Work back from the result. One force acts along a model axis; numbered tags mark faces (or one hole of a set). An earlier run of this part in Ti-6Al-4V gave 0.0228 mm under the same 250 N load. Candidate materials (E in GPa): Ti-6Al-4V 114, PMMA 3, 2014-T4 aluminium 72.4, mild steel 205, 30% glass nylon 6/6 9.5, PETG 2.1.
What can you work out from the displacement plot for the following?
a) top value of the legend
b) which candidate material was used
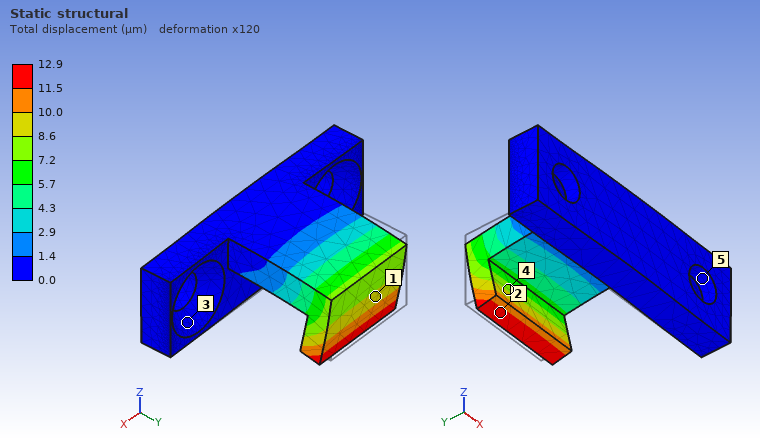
12.9 µm
mild steel
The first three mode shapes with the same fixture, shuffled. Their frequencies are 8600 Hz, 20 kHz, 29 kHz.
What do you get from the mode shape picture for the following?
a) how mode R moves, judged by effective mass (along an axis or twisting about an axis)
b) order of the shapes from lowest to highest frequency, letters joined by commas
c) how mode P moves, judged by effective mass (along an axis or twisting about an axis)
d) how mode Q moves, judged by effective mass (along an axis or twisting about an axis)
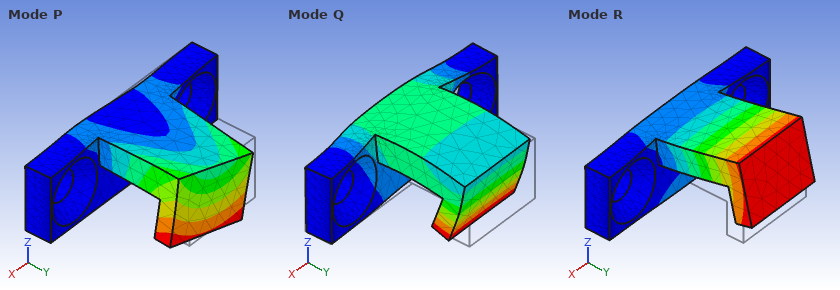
along Z
R, P, Q
along X
along Y
